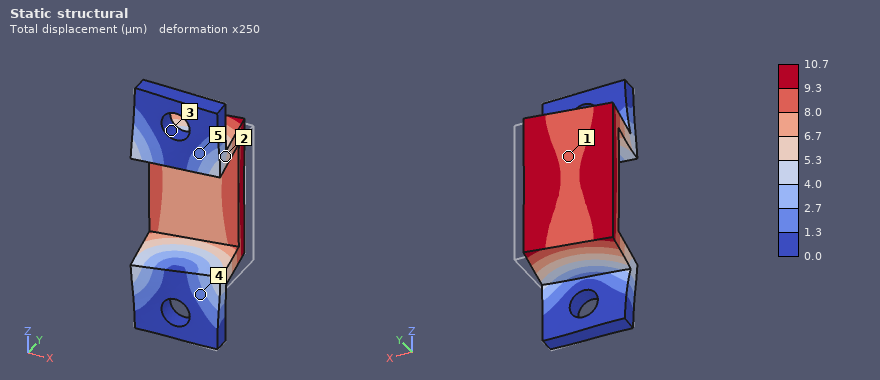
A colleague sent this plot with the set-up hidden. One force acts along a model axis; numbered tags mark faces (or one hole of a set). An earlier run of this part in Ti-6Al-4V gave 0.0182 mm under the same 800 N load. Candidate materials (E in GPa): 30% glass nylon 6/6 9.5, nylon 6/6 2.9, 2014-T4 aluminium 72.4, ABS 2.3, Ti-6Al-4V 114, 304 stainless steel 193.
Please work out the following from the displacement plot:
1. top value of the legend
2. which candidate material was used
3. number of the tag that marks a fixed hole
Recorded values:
10.7 µm
304 stainless steel
3
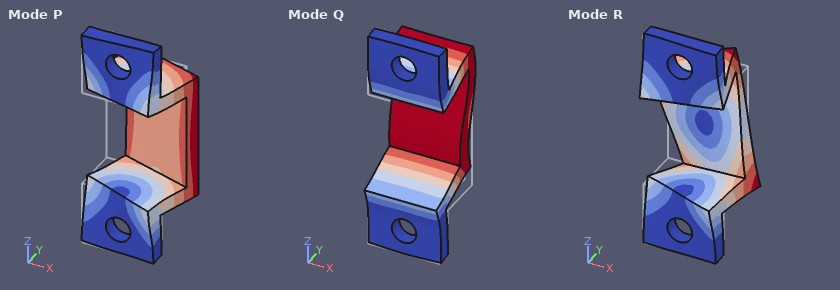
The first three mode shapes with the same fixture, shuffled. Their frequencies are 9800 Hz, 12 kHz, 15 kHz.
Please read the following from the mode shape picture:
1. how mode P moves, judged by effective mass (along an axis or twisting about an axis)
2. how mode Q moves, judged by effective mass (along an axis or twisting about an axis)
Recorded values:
along X
along Z
